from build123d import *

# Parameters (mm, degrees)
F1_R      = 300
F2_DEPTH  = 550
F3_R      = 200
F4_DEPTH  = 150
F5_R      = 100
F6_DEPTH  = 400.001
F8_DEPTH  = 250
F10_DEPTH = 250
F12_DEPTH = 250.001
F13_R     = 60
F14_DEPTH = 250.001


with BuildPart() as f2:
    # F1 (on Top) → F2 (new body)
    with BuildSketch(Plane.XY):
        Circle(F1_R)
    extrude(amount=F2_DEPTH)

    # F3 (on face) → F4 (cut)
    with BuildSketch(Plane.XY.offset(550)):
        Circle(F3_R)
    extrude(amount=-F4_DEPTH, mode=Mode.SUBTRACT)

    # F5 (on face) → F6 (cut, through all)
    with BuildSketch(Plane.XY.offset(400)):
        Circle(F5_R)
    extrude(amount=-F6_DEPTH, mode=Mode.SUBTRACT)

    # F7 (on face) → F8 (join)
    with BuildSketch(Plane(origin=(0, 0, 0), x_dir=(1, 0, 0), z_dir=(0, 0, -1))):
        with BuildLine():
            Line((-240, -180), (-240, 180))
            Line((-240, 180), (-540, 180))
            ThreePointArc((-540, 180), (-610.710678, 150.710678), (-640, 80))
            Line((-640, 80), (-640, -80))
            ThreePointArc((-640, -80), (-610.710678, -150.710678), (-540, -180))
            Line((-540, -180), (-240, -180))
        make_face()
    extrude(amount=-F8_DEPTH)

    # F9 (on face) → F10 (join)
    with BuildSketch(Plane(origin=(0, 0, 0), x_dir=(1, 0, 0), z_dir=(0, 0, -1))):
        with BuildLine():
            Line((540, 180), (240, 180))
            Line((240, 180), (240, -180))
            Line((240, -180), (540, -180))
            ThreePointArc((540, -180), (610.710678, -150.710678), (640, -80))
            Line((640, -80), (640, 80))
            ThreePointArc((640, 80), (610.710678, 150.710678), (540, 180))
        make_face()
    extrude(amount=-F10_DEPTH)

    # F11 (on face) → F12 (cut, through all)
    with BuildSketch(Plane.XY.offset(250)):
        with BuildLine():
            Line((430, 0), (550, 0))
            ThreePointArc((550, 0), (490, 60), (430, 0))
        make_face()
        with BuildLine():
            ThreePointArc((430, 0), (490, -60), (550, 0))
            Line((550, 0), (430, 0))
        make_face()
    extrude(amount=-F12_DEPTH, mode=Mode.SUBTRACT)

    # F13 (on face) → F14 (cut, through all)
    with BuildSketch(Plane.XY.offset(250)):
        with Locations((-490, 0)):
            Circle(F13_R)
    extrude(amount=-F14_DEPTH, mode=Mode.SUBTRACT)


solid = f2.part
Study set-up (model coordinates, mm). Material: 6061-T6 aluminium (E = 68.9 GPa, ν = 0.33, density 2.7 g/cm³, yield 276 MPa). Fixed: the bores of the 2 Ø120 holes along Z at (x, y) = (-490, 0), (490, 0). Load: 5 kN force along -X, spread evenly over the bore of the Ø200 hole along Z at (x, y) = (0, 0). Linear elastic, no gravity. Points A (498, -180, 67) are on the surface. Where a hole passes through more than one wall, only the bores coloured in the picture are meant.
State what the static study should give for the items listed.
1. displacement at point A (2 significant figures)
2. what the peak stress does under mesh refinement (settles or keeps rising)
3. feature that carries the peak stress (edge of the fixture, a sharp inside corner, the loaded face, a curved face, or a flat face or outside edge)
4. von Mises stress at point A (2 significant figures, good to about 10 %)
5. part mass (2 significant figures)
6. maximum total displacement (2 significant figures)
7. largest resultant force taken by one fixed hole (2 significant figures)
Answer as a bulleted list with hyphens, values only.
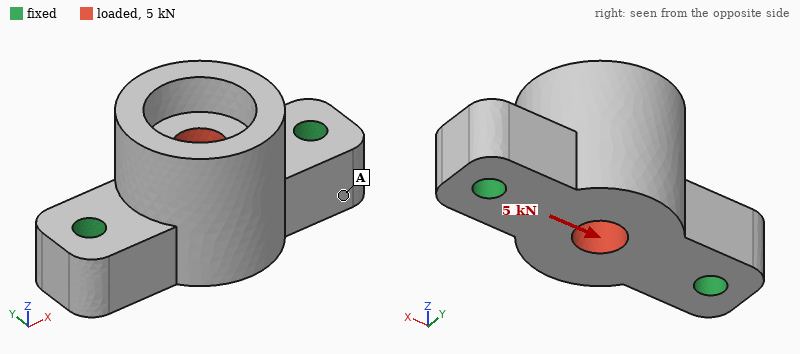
- 0.052 µm
- keeps rising
- edge of the fixture
- 0.0095 MPa
- 490 kg
- 0.24 µm
- 2.5 kN
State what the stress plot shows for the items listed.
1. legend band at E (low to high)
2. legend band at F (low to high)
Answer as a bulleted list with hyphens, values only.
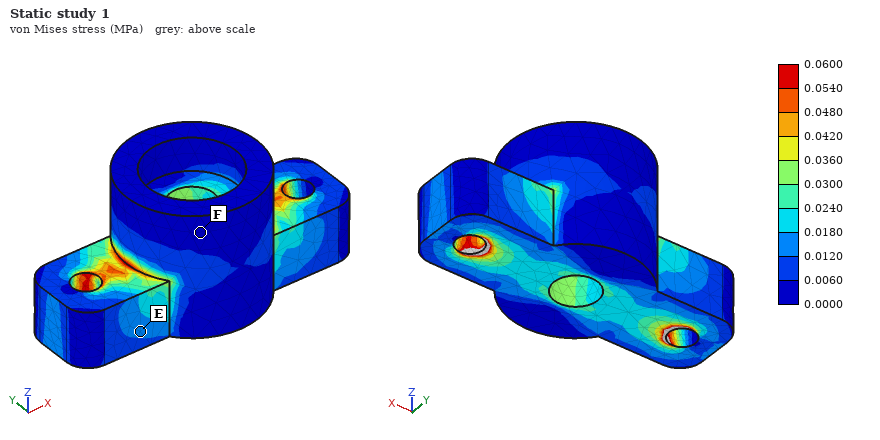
- 0.0120 to 0.0180 MPa
- 0.0000 to 0.0060 MPa
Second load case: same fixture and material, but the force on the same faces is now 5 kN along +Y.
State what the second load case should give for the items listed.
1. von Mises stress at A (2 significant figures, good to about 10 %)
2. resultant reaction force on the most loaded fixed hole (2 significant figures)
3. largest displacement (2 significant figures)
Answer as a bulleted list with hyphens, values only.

- 0.027 MPa
- 2.5 kN
- 1.4 µm
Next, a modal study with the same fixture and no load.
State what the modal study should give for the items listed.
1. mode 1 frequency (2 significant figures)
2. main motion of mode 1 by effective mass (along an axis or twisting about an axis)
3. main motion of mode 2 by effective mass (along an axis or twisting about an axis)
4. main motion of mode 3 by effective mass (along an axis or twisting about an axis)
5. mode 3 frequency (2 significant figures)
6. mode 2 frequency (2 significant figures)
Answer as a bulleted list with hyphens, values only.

- 460 Hz
- along Y
- along Z
- along Y
- 1000 Hz
- 790 Hz
